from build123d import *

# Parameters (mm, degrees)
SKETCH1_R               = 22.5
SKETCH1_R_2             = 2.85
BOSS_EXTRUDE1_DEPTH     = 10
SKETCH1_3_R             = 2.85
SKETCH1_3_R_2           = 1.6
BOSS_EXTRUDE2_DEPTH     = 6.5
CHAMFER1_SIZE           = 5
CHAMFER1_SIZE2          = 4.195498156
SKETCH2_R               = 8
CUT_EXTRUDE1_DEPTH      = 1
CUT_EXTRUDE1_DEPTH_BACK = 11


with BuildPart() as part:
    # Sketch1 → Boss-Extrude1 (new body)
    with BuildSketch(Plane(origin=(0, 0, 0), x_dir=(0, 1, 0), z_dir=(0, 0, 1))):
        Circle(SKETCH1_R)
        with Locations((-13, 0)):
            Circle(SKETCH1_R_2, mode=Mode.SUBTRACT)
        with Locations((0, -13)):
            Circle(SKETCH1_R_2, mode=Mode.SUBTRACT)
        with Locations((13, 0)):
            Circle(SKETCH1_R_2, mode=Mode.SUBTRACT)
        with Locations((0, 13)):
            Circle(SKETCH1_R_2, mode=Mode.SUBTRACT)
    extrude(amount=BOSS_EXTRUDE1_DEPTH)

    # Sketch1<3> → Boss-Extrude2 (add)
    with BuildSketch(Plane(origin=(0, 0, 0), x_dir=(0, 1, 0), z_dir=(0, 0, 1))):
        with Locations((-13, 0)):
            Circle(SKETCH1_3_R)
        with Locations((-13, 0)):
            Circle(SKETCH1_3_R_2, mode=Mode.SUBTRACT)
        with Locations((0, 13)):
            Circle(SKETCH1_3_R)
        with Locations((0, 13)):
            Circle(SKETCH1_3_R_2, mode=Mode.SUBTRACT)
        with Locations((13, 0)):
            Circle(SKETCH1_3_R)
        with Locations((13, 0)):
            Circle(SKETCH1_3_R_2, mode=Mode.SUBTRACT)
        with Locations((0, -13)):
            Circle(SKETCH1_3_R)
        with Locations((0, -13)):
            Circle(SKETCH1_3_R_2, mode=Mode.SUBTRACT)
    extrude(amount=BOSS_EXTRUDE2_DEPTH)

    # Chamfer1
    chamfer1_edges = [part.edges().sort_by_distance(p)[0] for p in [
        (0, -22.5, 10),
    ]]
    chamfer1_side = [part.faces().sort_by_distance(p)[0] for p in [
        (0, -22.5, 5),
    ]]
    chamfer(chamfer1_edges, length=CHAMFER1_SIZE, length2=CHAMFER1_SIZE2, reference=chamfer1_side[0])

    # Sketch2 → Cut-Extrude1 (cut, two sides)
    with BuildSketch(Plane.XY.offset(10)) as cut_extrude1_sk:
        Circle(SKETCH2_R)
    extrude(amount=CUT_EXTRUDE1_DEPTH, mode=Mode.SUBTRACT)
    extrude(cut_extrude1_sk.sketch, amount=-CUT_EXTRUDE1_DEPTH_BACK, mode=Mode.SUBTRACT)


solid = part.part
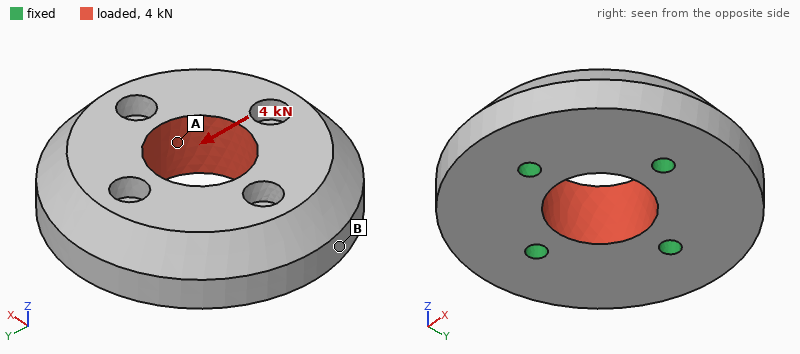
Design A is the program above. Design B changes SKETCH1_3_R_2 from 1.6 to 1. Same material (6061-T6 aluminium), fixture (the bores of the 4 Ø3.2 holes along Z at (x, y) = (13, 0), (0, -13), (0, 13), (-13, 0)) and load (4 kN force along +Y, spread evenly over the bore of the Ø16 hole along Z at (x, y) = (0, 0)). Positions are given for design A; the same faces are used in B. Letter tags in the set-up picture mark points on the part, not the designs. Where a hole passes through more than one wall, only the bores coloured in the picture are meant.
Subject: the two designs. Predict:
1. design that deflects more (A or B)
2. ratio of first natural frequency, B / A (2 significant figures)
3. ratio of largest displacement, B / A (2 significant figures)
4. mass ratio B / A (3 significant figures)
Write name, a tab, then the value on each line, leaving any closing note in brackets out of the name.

design that deflects more	B
ratio of first natural frequency, B / A	0.89
ratio of largest displacement, B / A	1.2
mass ratio B / A	1.01
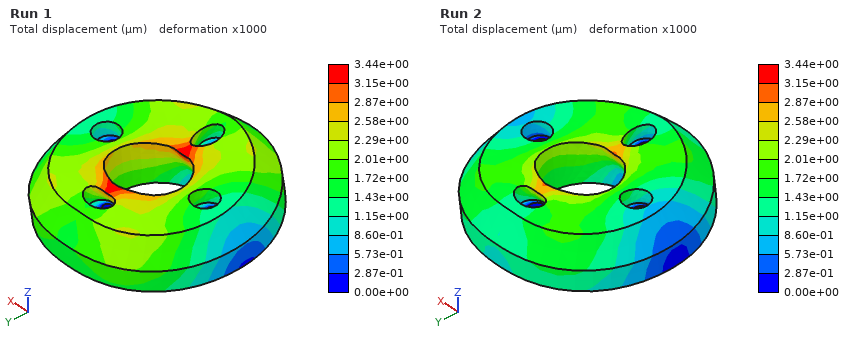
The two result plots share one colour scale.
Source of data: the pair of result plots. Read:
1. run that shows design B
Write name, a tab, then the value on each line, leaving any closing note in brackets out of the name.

run that shows design B	Run 1
